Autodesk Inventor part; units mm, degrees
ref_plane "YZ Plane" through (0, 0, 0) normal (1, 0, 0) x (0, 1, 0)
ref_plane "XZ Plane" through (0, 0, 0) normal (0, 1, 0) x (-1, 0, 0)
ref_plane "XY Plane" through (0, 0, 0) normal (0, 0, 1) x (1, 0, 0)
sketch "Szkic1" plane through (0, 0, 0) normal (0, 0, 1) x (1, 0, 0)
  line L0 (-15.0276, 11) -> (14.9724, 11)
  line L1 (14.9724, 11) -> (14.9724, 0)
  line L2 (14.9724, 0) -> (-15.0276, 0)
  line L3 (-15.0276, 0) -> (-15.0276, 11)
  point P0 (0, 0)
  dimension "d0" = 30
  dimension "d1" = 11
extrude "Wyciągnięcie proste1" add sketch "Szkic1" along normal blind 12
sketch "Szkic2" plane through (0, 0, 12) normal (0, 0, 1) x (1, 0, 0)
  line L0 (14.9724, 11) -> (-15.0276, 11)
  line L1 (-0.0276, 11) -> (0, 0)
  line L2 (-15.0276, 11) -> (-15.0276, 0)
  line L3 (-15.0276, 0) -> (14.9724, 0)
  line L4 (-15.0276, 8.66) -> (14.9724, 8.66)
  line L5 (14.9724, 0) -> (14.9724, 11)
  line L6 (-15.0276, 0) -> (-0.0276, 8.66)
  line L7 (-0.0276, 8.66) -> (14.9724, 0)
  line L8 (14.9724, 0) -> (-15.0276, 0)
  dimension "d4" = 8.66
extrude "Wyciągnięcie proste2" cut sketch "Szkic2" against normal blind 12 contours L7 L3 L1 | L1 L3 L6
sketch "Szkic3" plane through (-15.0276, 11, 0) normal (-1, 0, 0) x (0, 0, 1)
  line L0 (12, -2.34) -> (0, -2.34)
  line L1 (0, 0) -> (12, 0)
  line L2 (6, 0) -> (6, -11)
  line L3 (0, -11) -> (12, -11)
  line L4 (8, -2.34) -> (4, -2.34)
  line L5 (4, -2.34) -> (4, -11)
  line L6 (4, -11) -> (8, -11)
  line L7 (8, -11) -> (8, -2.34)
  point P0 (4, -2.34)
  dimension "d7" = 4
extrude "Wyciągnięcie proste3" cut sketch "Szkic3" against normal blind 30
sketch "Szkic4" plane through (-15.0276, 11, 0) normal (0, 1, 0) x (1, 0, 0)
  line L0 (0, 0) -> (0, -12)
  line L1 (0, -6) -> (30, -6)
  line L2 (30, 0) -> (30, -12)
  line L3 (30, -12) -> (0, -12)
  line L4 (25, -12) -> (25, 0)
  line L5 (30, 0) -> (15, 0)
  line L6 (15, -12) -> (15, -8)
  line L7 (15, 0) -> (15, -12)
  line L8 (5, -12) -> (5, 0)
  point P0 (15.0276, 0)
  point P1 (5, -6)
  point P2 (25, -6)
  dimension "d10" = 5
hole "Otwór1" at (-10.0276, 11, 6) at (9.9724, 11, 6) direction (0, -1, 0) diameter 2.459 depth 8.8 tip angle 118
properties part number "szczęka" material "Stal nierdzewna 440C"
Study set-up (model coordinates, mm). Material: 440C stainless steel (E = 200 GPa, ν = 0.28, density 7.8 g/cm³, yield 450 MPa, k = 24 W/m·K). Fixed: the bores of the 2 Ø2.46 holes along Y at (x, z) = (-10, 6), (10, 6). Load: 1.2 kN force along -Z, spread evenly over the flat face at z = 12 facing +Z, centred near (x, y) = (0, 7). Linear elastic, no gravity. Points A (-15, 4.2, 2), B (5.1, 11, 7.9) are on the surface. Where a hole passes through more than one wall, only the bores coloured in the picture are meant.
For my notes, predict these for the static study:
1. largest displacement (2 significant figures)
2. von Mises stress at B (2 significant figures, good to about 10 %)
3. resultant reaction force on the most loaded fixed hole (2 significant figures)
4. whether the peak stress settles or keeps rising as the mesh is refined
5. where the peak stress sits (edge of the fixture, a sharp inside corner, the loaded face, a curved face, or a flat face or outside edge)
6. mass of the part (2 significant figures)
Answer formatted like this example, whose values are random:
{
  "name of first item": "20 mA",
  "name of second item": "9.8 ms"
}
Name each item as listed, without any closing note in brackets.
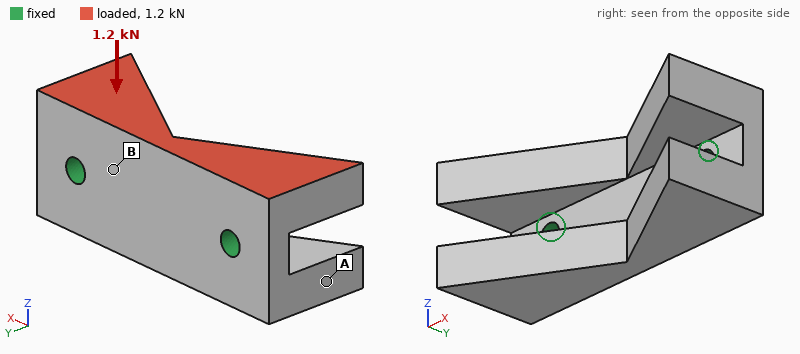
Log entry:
{
  "largest displacement": "23 µm",
  "von Mises stress at B": "52 MPa",
  "resultant reaction force on the most loaded fixed hole": "600 N",
  "whether the peak stress settles or keeps rising as the mesh is refined": "keeps rising",
  "where the peak stress sits": "edge of the fixture",
  "mass of the part": "15 g"
}
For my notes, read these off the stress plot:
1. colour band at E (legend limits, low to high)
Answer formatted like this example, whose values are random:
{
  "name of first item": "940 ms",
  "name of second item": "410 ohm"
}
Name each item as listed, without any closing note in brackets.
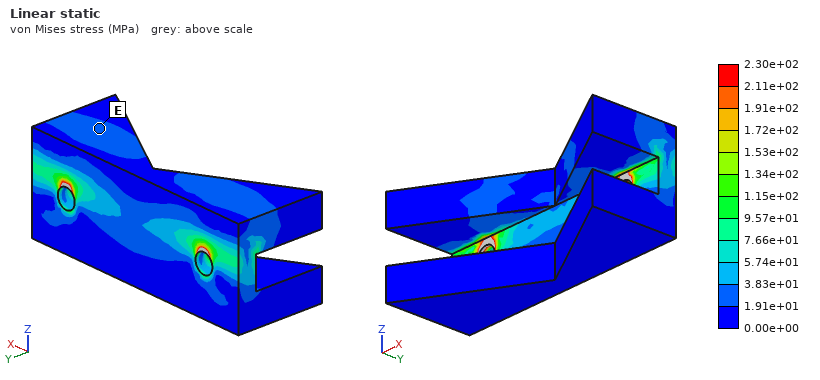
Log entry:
{
  "colour band at E": "1.91e+01 to 3.83e+01 MPa"
}
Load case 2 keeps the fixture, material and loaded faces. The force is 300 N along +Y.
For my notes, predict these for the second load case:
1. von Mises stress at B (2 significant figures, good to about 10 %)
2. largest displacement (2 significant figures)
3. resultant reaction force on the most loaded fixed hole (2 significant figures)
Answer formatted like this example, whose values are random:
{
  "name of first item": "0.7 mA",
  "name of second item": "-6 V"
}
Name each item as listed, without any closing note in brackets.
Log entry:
{
  "von Mises stress at B": "24 MPa",
  "largest displacement": "9.0 µm",
  "resultant reaction force on the most loaded fixed hole": "150 N"
}
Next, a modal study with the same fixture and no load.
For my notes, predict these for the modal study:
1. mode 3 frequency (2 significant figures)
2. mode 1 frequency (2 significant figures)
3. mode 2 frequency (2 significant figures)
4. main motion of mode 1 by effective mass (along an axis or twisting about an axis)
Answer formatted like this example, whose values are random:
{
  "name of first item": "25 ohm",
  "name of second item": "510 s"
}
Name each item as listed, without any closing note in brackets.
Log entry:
{
  "mode 3 frequency": "20 kHz",
  "mode 1 frequency": "15 kHz",
  "mode 2 frequency": "19 kHz",
  "main motion of mode 1 by effective mass": "along Z"
}
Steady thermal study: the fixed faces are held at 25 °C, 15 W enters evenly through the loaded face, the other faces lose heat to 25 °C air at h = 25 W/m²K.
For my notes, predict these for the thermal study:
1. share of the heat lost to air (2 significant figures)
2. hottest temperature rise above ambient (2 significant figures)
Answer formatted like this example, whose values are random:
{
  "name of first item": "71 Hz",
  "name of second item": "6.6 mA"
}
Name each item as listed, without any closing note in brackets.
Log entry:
{
  "share of the heat lost to air": "5.9 %",
  "hottest temperature rise above ambient": "63 K"
}
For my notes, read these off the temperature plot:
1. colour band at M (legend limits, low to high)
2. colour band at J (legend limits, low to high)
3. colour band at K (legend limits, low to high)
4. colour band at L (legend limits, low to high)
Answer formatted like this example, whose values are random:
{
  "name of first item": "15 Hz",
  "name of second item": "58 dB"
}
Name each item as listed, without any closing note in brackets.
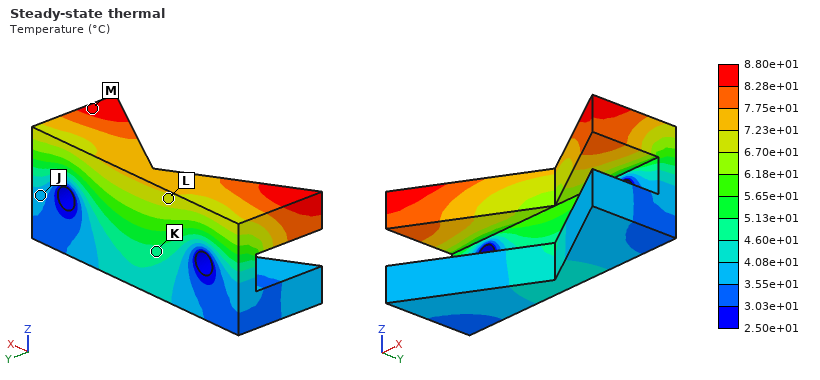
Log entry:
{
  "colour band at M": "8.28e+01 to 8.80e+01 °C",
  "colour band at J": "3.55e+01 to 4.08e+01 °C",
  "colour band at K": "4.60e+01 to 5.13e+01 °C",
  "colour band at L": "6.70e+01 to 7.23e+01 °C"
}
